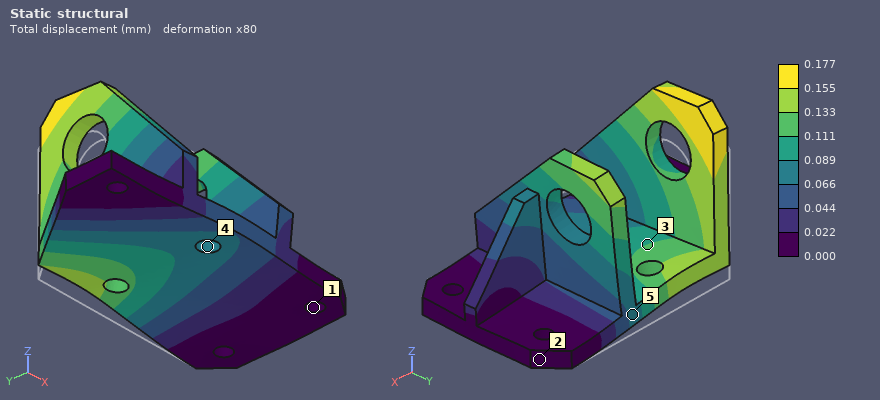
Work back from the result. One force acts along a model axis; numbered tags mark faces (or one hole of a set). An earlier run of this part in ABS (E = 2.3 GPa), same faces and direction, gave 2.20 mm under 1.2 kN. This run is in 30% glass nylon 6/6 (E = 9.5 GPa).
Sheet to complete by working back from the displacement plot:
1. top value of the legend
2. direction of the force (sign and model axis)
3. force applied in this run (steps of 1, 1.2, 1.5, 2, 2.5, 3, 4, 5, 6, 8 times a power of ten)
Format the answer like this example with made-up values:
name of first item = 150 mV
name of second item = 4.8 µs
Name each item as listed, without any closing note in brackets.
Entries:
top value of the legend = 0.177 mm
direction of the force = +Z
force applied in this run = 400 N
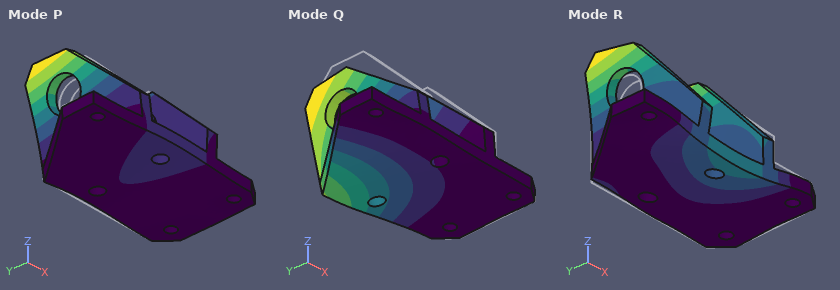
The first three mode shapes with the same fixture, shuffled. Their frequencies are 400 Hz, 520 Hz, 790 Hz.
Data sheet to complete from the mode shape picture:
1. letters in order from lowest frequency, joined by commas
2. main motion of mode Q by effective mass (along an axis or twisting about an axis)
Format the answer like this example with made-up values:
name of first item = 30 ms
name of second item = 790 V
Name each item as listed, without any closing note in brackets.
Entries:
letters in order from lowest frequency, joined by commas = Q, P, R
main motion of mode Q by effective mass = along Z
